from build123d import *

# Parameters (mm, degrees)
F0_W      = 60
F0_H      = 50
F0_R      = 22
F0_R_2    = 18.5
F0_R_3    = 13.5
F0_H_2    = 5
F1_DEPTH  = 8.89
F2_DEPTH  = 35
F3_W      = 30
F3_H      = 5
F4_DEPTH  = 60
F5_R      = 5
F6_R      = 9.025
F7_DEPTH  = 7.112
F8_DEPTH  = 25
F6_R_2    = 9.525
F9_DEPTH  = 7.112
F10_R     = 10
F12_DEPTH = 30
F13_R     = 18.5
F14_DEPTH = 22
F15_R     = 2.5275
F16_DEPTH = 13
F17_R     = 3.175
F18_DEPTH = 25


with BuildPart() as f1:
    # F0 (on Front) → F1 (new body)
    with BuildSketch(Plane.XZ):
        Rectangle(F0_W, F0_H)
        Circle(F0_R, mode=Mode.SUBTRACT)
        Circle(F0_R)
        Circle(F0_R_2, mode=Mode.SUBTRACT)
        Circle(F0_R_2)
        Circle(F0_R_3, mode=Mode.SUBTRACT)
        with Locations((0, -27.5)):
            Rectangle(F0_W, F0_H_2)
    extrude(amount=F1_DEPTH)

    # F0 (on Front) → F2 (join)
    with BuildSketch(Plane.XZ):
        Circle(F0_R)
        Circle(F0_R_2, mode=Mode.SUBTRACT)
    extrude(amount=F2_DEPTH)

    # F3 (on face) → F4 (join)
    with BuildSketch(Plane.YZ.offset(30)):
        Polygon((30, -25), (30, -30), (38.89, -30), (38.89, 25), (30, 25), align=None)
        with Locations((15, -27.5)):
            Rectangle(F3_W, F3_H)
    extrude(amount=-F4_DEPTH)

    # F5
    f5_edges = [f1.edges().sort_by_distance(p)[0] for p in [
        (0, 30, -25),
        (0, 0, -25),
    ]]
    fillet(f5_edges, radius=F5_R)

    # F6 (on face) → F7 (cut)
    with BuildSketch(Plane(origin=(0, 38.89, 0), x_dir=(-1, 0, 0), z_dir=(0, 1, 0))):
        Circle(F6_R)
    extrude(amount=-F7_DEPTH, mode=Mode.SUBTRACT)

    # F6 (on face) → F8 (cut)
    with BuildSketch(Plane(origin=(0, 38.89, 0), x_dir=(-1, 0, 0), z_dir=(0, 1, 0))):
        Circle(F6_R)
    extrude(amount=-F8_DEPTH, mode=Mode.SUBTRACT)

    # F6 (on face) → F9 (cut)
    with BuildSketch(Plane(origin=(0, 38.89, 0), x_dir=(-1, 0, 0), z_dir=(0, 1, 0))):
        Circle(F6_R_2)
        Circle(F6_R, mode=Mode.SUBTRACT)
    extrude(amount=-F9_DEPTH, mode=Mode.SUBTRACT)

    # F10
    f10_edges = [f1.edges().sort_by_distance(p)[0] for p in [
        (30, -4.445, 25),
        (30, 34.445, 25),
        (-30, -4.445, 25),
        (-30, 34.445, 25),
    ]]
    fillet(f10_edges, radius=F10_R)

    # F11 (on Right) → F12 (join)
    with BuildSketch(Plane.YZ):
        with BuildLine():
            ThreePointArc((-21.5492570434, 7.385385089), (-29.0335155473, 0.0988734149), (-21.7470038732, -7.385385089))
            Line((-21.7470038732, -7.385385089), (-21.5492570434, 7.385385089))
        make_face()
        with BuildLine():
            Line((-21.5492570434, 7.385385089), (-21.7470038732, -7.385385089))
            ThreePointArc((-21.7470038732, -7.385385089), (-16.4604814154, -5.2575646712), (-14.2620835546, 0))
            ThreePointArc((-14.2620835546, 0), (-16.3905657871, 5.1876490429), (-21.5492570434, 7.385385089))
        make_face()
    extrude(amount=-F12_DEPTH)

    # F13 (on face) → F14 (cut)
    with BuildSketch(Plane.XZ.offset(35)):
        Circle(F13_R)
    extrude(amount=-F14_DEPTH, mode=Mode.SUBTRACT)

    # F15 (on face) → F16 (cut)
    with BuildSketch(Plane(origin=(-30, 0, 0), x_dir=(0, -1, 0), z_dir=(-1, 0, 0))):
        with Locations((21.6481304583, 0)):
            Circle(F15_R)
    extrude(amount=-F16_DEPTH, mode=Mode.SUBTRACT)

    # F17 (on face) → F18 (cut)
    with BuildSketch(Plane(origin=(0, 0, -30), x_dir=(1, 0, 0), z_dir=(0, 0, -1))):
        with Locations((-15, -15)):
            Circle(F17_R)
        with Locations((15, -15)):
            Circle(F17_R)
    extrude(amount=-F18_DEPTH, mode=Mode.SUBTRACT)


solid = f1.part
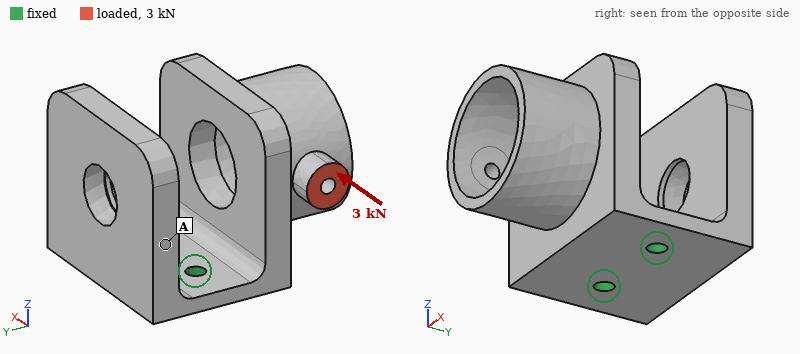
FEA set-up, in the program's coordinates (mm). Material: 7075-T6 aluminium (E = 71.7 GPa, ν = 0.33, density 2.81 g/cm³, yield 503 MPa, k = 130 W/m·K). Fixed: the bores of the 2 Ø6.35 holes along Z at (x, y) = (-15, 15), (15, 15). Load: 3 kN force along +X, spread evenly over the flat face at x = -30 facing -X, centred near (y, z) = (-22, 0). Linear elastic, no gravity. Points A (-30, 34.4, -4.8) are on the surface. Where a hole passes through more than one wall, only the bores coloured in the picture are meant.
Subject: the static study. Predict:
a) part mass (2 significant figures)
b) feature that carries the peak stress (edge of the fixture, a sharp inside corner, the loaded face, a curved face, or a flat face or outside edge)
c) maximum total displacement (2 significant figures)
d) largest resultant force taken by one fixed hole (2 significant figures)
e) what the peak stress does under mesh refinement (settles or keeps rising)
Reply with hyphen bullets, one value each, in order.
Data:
- 200 g
- edge of the fixture
- 0.22 mm
- 4.3 kN
- keeps rising
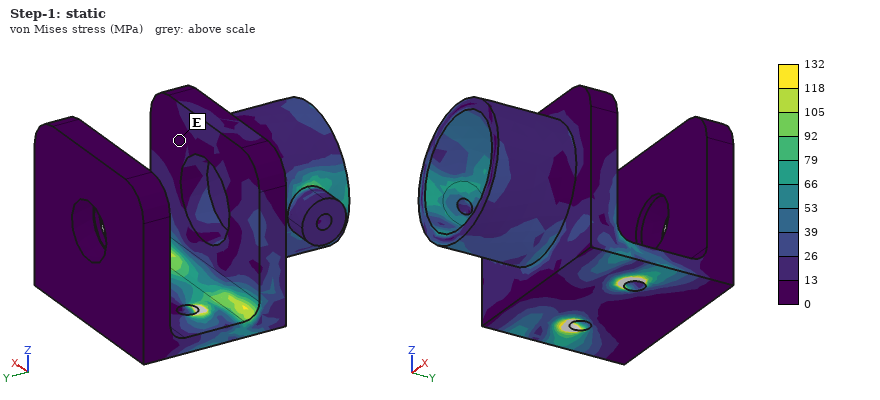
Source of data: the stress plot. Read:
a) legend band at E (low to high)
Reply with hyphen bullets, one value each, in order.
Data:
- 0 to 13 MPa
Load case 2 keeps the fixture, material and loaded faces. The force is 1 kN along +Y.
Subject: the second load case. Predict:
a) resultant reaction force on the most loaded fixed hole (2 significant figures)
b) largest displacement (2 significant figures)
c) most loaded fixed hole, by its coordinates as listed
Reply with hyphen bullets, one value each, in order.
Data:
- 1.4 kN
- 0.58 mm
- (-15, 15)
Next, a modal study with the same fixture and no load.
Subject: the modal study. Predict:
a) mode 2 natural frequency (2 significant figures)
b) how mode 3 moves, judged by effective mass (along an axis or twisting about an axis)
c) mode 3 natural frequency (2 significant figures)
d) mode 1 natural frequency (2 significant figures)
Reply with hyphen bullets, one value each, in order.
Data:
- 1000 Hz
- along X
- 2100 Hz
- 750 Hz
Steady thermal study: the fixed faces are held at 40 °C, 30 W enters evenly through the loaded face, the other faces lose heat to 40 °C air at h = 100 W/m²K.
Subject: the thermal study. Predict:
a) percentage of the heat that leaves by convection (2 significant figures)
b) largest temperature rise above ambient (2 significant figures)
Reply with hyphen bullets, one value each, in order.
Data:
- 60 %
- 41 K
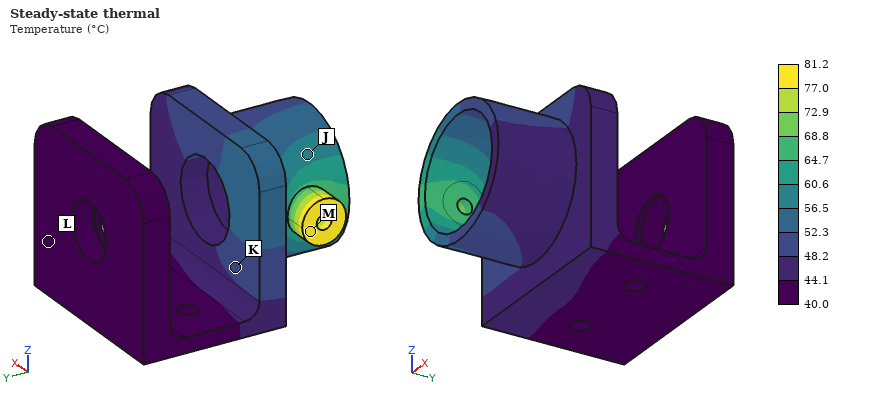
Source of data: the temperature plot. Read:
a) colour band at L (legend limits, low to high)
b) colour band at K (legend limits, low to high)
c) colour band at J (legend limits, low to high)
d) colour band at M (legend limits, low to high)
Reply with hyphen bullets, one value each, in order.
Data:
- 40.0 to 44.1 °C
- 48.2 to 52.3 °C
- 56.5 to 60.6 °C
- 77.0 to 81.2 °C
